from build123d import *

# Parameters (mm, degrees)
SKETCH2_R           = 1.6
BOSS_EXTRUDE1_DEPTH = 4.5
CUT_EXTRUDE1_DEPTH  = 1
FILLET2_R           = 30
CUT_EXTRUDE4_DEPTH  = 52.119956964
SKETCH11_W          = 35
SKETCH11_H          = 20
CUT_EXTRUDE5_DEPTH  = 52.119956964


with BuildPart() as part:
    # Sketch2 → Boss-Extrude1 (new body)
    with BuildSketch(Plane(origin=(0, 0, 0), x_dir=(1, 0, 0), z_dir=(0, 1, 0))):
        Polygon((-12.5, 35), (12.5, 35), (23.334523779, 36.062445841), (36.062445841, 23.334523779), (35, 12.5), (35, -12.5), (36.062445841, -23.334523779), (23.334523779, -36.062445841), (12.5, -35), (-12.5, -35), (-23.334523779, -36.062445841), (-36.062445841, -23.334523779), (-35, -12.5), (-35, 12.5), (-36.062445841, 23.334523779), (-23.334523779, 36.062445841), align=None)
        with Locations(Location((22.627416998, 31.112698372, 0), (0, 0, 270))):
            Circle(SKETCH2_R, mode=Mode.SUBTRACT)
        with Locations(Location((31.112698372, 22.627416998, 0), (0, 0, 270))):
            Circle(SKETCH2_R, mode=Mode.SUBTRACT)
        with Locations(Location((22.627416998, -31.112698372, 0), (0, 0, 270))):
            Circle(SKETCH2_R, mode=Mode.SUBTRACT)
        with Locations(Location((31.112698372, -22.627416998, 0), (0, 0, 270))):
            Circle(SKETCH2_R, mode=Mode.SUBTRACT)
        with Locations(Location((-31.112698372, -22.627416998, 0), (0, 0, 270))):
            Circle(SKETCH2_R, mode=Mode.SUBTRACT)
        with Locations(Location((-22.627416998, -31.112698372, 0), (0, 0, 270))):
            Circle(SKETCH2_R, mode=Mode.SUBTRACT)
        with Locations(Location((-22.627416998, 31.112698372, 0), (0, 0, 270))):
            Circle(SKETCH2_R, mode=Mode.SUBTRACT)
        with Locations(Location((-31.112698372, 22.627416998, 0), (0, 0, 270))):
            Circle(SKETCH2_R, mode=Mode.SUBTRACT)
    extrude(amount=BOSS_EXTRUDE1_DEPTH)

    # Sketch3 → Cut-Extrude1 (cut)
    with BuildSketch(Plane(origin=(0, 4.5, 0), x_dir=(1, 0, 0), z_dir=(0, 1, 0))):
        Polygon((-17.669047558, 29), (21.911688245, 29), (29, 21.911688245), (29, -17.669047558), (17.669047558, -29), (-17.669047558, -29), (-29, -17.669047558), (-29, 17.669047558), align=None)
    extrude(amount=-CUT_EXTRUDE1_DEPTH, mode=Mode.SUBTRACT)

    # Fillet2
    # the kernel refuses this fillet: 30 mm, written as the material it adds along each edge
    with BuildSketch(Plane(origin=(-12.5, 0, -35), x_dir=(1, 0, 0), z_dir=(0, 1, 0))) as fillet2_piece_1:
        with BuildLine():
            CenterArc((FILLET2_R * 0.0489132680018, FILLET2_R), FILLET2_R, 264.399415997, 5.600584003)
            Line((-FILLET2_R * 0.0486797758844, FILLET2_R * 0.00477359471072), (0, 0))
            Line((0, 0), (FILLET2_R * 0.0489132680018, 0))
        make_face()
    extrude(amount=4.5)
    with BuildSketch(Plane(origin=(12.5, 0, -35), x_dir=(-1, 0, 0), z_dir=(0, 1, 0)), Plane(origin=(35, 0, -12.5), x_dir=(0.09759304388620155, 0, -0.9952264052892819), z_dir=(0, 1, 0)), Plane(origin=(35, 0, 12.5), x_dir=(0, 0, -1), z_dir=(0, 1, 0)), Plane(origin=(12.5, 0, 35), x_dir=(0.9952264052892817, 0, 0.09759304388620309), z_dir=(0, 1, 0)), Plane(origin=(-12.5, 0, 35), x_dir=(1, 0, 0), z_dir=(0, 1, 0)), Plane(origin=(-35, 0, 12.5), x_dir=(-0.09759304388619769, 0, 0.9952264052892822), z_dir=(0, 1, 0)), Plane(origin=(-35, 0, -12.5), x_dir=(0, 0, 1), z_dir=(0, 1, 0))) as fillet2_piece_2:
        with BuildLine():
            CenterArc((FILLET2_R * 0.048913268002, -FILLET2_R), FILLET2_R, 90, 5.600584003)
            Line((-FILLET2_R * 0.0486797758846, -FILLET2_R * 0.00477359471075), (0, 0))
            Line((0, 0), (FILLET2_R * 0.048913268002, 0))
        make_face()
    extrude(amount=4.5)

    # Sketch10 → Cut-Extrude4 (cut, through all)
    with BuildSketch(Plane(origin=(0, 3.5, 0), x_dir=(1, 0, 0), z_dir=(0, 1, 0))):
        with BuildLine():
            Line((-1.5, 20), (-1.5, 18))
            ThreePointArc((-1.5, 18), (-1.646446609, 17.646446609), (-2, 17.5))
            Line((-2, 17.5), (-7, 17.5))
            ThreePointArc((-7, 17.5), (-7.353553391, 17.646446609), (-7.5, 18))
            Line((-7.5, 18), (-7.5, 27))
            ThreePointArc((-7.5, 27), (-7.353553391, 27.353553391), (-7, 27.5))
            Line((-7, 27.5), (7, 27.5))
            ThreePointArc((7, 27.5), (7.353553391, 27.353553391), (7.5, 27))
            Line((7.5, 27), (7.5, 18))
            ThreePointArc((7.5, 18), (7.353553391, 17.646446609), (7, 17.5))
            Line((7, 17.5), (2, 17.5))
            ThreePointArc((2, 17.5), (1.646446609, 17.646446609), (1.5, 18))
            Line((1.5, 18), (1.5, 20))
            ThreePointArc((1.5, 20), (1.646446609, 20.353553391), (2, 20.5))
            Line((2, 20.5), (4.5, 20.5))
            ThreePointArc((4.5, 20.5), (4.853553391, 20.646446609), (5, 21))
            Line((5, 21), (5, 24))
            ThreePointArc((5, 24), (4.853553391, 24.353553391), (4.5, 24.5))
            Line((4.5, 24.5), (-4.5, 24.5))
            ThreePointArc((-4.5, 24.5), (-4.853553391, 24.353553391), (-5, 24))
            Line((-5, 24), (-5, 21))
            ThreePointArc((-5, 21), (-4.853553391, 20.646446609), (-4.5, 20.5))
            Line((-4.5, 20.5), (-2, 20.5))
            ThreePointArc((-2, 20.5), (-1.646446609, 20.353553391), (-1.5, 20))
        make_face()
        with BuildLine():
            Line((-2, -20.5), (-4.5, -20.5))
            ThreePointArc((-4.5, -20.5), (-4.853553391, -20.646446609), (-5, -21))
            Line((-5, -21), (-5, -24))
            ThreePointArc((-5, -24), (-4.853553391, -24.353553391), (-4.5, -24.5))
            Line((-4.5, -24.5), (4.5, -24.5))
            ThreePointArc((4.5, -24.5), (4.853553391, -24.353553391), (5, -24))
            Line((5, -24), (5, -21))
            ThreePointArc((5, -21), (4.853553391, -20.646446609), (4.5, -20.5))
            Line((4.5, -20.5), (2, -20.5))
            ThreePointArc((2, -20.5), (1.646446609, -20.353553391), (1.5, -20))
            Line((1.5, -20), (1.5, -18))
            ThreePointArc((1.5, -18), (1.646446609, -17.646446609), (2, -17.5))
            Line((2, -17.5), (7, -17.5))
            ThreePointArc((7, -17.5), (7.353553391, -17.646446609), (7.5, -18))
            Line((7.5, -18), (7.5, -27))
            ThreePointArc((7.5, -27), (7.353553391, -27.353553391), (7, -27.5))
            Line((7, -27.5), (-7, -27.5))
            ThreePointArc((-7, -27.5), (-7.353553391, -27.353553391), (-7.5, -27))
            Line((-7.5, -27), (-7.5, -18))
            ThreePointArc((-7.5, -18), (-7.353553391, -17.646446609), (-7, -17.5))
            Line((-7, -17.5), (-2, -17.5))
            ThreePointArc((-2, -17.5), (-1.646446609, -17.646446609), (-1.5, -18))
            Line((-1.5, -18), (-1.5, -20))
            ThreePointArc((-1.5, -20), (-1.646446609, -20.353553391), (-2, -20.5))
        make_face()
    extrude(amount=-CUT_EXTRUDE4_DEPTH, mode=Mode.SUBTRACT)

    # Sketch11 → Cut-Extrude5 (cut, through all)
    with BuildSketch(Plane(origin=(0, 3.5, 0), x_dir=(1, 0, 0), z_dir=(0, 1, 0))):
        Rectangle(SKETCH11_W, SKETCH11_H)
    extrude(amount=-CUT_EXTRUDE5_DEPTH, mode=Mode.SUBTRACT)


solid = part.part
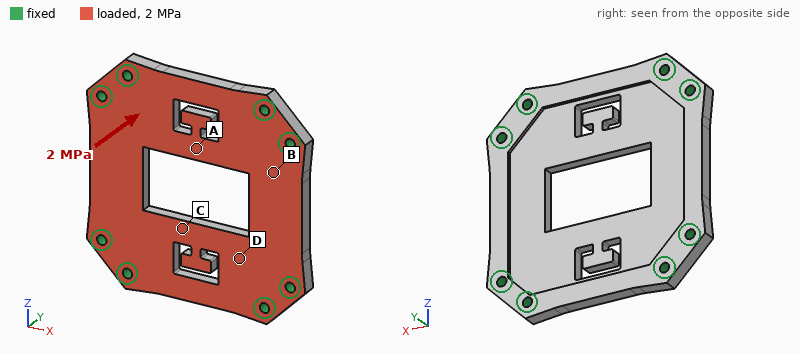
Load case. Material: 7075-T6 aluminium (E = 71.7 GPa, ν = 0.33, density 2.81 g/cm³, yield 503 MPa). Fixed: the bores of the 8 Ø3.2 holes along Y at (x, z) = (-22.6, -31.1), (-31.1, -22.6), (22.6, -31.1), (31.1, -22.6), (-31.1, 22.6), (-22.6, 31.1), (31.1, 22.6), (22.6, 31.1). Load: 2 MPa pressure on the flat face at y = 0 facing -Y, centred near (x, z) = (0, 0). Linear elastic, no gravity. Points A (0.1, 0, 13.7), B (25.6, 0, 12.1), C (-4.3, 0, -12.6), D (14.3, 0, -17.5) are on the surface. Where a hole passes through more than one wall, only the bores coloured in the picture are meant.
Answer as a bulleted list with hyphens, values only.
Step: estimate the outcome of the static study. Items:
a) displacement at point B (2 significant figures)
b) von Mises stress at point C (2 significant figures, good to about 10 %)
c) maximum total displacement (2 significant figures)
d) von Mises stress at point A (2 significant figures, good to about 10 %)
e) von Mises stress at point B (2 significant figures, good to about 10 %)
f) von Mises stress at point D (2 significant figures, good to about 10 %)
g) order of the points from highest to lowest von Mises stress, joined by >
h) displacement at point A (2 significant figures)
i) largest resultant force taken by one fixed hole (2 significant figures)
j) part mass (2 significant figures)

- 0.067 mm
- 99 MPa
- 0.25 mm
- 130 MPa
- 52 MPa
- 27 MPa
- A > C > B > D
- 0.21 mm
- 990 N
- 41 g
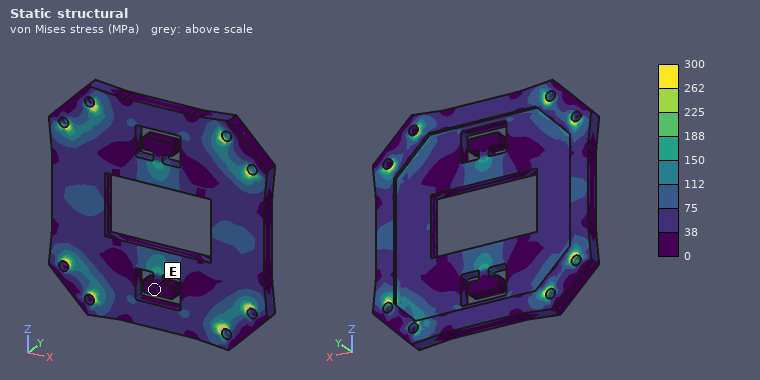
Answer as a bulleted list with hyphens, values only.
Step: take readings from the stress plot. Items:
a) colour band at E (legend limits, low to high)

- 0 to 38 MPa
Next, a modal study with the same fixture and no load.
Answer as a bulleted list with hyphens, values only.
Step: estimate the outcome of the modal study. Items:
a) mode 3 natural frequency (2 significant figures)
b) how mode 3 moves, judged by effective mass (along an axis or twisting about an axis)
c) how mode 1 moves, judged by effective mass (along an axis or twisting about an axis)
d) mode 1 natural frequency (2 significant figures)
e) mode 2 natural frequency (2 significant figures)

- 9500 Hz
- twisting about Z
- along Y
- 6200 Hz
- 7400 Hz
